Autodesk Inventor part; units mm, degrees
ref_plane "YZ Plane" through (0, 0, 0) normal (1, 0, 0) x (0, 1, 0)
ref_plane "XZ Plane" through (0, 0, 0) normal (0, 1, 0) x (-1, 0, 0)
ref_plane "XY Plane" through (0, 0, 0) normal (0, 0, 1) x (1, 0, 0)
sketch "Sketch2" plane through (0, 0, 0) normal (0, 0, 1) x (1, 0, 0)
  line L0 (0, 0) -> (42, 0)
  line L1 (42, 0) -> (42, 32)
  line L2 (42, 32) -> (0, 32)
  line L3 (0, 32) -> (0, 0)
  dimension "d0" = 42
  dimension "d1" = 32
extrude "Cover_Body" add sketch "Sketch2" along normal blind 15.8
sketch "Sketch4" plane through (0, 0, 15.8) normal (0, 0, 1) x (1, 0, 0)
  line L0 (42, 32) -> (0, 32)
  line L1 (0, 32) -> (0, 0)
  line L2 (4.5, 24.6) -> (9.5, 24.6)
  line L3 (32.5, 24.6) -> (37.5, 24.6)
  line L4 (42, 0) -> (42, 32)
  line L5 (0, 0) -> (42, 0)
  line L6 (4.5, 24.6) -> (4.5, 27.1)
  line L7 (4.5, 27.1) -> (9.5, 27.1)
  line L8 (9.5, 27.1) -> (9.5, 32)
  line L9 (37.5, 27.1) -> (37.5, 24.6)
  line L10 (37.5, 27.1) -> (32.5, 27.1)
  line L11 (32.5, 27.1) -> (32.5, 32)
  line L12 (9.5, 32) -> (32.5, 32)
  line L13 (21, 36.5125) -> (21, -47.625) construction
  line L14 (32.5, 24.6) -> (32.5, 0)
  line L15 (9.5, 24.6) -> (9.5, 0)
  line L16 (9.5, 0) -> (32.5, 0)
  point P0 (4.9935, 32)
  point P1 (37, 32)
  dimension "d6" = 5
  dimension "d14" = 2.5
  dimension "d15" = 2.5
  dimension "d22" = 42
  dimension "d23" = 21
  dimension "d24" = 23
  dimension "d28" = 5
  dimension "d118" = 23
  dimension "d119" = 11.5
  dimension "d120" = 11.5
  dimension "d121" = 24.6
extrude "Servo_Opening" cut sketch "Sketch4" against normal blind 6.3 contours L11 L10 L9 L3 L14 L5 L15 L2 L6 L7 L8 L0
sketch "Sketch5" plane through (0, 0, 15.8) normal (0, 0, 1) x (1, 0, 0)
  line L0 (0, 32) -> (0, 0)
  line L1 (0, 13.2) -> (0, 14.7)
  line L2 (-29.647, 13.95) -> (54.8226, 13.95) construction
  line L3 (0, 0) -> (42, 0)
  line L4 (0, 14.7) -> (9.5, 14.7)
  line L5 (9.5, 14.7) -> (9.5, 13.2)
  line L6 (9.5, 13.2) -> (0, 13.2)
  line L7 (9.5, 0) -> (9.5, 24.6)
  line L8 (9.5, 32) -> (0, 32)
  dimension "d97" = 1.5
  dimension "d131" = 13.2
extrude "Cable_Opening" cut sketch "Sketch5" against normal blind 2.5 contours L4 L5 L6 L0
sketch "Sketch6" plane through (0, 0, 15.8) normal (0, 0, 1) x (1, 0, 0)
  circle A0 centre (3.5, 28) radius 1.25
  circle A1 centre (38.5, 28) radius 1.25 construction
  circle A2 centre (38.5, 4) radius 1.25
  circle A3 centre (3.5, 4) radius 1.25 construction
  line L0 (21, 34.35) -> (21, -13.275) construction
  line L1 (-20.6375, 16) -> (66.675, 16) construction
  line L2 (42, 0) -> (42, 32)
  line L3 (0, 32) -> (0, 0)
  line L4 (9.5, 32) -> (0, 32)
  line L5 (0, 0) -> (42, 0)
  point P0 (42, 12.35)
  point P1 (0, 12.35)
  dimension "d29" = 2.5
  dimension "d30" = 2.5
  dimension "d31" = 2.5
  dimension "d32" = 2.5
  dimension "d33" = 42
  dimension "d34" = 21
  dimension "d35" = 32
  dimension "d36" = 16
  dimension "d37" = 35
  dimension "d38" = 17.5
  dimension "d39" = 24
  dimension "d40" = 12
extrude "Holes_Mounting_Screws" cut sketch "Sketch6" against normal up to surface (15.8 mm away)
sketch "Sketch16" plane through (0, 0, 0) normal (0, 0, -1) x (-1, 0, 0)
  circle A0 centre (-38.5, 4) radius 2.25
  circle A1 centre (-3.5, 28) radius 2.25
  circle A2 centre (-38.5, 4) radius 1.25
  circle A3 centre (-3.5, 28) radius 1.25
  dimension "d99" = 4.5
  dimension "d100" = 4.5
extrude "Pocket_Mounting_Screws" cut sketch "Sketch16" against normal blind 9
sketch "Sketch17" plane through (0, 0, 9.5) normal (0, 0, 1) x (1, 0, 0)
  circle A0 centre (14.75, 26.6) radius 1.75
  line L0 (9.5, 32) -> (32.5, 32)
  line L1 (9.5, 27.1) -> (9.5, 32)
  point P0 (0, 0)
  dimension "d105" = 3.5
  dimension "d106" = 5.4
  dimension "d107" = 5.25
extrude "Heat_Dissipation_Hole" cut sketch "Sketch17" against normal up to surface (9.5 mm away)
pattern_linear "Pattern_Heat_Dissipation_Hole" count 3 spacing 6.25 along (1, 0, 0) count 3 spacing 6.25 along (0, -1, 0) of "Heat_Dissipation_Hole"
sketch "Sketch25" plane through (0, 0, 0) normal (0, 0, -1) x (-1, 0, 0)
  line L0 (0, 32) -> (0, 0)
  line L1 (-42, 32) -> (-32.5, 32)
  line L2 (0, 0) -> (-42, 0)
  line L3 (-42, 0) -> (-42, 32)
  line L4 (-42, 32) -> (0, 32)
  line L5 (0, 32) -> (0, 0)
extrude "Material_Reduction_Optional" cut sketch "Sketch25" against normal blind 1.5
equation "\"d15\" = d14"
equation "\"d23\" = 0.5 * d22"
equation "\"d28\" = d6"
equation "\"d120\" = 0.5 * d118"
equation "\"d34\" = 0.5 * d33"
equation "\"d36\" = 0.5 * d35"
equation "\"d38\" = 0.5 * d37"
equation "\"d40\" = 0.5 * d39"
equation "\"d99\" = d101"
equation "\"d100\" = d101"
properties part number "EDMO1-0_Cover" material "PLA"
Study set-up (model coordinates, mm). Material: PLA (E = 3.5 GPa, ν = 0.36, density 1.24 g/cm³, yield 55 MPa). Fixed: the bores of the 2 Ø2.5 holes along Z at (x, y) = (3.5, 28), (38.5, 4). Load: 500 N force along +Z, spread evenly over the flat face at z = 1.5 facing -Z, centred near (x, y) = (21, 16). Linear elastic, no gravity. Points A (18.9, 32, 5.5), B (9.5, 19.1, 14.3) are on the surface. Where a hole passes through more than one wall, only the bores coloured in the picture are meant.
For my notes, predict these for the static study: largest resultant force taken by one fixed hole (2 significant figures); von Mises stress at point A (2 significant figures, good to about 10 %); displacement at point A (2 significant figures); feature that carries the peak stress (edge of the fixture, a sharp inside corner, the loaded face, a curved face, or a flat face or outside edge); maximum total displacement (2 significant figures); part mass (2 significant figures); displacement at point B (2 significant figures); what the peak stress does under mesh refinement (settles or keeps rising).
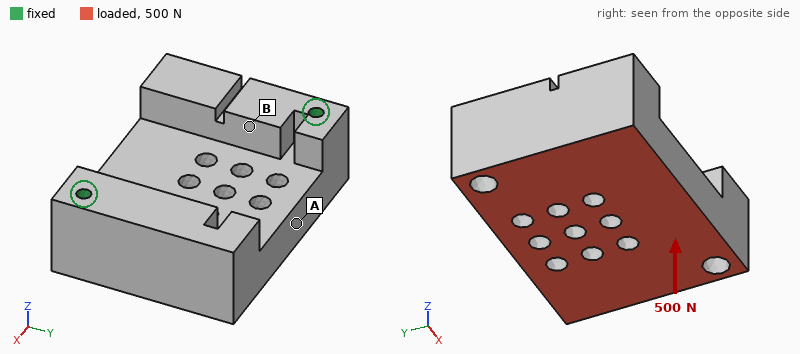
330 N
5.1 MPa
0.045 mm
edge of the fixture
0.12 mm
17 g
0.047 mm
keeps rising
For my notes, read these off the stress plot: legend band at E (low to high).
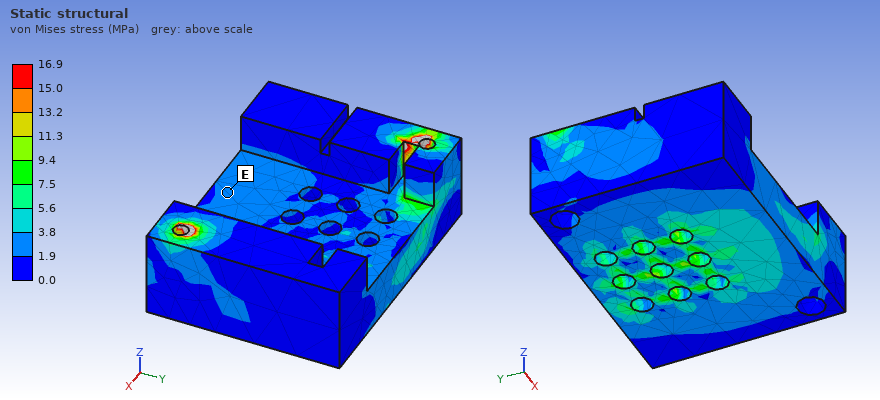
1.9 to 3.8 MPa
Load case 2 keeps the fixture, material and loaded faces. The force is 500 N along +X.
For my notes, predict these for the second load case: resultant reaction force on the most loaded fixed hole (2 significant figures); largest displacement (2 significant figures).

280 N
0.18 mm
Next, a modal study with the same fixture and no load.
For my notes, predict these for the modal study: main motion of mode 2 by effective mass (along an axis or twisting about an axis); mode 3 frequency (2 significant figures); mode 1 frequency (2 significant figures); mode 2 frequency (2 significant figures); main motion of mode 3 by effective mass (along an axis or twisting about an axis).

along Z
5000 Hz
2000 Hz
3300 Hz
along X
